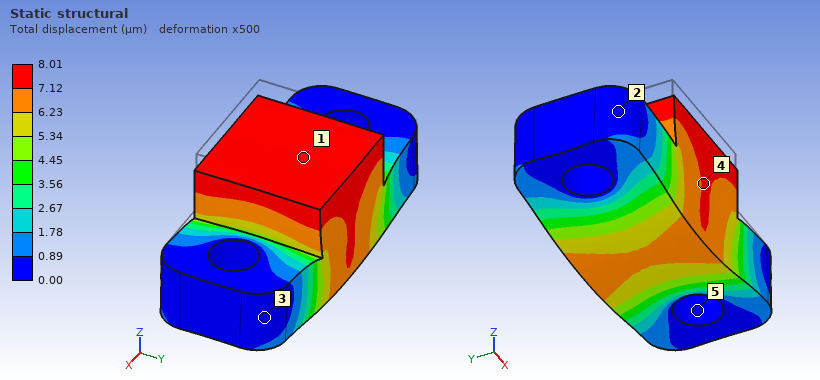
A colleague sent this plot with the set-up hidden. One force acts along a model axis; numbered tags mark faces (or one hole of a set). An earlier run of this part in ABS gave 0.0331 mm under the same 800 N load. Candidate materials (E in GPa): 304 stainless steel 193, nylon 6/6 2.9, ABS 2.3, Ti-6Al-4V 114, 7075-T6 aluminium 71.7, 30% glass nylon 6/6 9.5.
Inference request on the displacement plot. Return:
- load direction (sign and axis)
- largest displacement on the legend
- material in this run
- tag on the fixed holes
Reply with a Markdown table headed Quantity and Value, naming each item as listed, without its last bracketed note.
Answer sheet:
| Quantity | Value |
|---|---|
| load direction | -Z |
| largest displacement on the legend | 8.01 µm |
| material in this run | 30% glass nylon 6/6 |
| tag on the fixed holes | 5 |
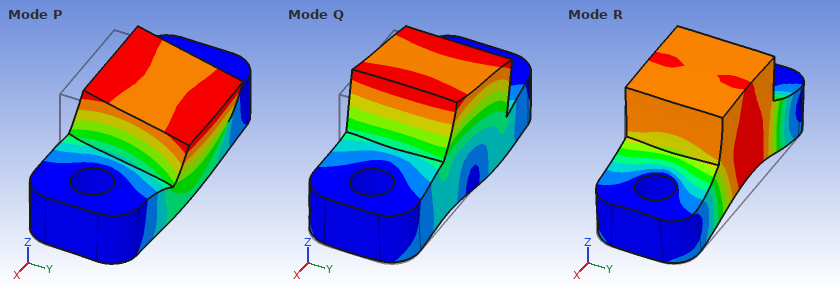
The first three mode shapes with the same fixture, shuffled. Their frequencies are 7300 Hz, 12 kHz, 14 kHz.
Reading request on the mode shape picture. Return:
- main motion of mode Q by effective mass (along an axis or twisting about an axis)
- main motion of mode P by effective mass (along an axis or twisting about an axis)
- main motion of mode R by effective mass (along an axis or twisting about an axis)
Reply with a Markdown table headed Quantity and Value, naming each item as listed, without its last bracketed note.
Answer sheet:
| Quantity | Value |
|---|---|
| main motion of mode Q by effective mass | along X |
| main motion of mode P by effective mass | along Y |
| main motion of mode R by effective mass | along Z |
